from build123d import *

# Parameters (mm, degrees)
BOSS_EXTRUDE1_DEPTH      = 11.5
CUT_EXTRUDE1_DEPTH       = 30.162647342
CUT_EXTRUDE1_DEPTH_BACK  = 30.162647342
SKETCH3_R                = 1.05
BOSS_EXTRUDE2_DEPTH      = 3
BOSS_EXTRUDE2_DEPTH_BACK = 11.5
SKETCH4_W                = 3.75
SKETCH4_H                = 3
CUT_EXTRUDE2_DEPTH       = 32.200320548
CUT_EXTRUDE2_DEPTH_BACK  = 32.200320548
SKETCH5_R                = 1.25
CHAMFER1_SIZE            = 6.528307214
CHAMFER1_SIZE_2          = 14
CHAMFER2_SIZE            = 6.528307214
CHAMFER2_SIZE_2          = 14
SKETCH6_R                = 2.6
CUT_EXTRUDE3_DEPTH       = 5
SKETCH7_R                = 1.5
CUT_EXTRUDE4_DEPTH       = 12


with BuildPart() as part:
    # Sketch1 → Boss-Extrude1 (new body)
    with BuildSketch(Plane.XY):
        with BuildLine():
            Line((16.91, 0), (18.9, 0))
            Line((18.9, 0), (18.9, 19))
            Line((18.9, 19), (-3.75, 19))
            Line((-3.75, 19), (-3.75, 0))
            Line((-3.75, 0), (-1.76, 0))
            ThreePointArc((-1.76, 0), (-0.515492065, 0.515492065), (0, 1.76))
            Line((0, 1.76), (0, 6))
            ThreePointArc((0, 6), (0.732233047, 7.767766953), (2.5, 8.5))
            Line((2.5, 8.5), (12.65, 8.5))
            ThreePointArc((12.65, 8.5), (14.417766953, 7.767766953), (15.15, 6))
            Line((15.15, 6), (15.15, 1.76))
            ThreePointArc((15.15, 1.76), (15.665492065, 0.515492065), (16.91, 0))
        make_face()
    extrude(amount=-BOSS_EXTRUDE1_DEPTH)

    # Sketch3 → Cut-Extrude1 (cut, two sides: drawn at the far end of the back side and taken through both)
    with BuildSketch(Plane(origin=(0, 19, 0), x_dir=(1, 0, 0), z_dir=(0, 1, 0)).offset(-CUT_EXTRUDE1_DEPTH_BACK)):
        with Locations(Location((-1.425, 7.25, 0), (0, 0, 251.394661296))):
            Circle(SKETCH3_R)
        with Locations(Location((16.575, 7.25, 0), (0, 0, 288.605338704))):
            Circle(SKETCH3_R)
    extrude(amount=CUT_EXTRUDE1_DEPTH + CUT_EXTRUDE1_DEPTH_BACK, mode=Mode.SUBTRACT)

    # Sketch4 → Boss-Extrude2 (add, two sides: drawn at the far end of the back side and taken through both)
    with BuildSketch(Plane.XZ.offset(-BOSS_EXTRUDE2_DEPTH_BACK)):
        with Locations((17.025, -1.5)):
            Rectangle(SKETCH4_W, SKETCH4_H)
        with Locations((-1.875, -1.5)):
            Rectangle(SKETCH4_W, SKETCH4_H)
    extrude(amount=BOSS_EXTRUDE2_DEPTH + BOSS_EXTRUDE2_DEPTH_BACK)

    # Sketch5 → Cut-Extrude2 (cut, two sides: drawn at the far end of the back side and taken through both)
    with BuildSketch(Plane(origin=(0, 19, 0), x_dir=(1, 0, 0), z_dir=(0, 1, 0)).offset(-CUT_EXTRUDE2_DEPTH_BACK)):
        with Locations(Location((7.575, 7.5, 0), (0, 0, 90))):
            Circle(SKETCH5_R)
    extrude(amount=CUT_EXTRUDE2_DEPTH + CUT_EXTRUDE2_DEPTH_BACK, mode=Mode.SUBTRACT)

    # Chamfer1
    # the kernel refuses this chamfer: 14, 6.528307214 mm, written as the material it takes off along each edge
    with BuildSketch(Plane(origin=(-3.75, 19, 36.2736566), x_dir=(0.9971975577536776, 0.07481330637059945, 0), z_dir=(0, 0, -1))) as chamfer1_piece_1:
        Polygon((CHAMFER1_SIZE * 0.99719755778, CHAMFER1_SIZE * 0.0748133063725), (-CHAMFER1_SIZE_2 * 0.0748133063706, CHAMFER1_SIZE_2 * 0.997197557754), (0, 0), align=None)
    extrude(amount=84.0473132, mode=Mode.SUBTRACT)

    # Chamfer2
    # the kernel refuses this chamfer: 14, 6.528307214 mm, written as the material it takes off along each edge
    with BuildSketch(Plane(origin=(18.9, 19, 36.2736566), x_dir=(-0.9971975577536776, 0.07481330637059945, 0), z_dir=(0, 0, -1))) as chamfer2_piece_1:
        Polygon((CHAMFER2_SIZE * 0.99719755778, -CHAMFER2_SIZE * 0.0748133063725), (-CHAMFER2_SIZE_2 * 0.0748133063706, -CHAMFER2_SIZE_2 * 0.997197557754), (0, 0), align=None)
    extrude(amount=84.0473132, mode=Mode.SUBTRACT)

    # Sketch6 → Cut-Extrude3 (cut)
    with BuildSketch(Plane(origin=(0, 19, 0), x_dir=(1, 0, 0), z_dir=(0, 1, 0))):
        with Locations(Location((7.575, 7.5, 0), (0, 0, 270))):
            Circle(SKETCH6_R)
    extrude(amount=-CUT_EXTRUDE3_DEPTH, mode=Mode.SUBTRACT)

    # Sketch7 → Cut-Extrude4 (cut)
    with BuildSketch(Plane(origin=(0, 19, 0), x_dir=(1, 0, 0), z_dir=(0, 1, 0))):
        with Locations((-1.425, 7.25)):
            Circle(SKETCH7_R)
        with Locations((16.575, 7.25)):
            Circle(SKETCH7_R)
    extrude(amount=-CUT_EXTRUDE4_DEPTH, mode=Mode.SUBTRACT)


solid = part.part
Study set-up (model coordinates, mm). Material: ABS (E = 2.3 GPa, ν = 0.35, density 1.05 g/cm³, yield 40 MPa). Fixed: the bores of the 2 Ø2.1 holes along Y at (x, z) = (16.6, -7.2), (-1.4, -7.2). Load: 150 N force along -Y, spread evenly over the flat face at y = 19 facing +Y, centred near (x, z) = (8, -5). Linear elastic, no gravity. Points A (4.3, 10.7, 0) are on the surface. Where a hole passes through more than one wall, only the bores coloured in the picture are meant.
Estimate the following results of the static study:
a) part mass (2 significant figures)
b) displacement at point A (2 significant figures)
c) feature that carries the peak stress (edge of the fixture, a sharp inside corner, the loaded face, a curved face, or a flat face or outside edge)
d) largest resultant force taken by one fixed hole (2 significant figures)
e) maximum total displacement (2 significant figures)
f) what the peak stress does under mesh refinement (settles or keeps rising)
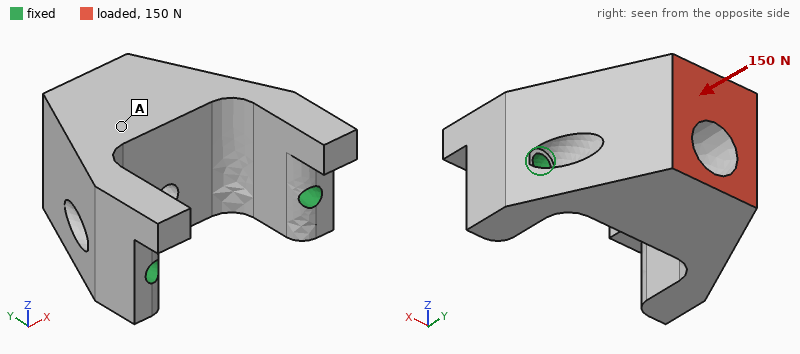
2.4 g
33 µm
edge of the fixture
81 N
46 µm
keeps rising
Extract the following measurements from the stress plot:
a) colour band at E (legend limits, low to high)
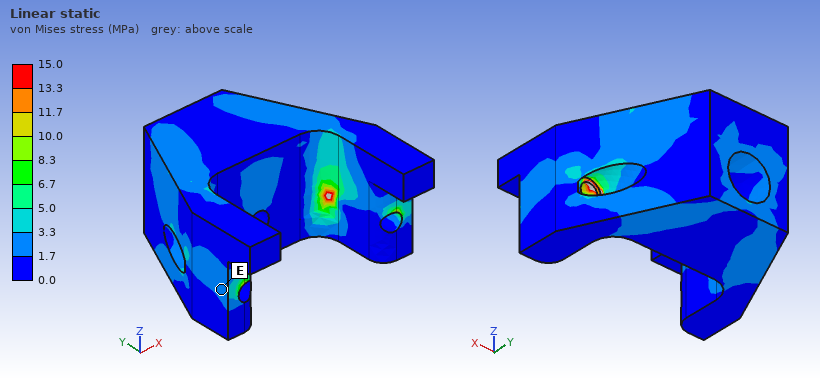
1.7 to 3.3 MPa
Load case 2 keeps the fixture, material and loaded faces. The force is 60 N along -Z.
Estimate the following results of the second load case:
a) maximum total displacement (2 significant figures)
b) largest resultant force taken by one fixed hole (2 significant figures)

0.13 mm
30 N
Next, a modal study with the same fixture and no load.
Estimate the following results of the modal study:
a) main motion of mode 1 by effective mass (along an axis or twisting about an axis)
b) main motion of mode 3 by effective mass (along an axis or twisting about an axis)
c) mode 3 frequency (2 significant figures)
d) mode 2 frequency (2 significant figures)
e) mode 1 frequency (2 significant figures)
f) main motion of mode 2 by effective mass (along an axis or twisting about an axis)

along Z
along Y
11 kHz
7800 Hz
4400 Hz
along X
